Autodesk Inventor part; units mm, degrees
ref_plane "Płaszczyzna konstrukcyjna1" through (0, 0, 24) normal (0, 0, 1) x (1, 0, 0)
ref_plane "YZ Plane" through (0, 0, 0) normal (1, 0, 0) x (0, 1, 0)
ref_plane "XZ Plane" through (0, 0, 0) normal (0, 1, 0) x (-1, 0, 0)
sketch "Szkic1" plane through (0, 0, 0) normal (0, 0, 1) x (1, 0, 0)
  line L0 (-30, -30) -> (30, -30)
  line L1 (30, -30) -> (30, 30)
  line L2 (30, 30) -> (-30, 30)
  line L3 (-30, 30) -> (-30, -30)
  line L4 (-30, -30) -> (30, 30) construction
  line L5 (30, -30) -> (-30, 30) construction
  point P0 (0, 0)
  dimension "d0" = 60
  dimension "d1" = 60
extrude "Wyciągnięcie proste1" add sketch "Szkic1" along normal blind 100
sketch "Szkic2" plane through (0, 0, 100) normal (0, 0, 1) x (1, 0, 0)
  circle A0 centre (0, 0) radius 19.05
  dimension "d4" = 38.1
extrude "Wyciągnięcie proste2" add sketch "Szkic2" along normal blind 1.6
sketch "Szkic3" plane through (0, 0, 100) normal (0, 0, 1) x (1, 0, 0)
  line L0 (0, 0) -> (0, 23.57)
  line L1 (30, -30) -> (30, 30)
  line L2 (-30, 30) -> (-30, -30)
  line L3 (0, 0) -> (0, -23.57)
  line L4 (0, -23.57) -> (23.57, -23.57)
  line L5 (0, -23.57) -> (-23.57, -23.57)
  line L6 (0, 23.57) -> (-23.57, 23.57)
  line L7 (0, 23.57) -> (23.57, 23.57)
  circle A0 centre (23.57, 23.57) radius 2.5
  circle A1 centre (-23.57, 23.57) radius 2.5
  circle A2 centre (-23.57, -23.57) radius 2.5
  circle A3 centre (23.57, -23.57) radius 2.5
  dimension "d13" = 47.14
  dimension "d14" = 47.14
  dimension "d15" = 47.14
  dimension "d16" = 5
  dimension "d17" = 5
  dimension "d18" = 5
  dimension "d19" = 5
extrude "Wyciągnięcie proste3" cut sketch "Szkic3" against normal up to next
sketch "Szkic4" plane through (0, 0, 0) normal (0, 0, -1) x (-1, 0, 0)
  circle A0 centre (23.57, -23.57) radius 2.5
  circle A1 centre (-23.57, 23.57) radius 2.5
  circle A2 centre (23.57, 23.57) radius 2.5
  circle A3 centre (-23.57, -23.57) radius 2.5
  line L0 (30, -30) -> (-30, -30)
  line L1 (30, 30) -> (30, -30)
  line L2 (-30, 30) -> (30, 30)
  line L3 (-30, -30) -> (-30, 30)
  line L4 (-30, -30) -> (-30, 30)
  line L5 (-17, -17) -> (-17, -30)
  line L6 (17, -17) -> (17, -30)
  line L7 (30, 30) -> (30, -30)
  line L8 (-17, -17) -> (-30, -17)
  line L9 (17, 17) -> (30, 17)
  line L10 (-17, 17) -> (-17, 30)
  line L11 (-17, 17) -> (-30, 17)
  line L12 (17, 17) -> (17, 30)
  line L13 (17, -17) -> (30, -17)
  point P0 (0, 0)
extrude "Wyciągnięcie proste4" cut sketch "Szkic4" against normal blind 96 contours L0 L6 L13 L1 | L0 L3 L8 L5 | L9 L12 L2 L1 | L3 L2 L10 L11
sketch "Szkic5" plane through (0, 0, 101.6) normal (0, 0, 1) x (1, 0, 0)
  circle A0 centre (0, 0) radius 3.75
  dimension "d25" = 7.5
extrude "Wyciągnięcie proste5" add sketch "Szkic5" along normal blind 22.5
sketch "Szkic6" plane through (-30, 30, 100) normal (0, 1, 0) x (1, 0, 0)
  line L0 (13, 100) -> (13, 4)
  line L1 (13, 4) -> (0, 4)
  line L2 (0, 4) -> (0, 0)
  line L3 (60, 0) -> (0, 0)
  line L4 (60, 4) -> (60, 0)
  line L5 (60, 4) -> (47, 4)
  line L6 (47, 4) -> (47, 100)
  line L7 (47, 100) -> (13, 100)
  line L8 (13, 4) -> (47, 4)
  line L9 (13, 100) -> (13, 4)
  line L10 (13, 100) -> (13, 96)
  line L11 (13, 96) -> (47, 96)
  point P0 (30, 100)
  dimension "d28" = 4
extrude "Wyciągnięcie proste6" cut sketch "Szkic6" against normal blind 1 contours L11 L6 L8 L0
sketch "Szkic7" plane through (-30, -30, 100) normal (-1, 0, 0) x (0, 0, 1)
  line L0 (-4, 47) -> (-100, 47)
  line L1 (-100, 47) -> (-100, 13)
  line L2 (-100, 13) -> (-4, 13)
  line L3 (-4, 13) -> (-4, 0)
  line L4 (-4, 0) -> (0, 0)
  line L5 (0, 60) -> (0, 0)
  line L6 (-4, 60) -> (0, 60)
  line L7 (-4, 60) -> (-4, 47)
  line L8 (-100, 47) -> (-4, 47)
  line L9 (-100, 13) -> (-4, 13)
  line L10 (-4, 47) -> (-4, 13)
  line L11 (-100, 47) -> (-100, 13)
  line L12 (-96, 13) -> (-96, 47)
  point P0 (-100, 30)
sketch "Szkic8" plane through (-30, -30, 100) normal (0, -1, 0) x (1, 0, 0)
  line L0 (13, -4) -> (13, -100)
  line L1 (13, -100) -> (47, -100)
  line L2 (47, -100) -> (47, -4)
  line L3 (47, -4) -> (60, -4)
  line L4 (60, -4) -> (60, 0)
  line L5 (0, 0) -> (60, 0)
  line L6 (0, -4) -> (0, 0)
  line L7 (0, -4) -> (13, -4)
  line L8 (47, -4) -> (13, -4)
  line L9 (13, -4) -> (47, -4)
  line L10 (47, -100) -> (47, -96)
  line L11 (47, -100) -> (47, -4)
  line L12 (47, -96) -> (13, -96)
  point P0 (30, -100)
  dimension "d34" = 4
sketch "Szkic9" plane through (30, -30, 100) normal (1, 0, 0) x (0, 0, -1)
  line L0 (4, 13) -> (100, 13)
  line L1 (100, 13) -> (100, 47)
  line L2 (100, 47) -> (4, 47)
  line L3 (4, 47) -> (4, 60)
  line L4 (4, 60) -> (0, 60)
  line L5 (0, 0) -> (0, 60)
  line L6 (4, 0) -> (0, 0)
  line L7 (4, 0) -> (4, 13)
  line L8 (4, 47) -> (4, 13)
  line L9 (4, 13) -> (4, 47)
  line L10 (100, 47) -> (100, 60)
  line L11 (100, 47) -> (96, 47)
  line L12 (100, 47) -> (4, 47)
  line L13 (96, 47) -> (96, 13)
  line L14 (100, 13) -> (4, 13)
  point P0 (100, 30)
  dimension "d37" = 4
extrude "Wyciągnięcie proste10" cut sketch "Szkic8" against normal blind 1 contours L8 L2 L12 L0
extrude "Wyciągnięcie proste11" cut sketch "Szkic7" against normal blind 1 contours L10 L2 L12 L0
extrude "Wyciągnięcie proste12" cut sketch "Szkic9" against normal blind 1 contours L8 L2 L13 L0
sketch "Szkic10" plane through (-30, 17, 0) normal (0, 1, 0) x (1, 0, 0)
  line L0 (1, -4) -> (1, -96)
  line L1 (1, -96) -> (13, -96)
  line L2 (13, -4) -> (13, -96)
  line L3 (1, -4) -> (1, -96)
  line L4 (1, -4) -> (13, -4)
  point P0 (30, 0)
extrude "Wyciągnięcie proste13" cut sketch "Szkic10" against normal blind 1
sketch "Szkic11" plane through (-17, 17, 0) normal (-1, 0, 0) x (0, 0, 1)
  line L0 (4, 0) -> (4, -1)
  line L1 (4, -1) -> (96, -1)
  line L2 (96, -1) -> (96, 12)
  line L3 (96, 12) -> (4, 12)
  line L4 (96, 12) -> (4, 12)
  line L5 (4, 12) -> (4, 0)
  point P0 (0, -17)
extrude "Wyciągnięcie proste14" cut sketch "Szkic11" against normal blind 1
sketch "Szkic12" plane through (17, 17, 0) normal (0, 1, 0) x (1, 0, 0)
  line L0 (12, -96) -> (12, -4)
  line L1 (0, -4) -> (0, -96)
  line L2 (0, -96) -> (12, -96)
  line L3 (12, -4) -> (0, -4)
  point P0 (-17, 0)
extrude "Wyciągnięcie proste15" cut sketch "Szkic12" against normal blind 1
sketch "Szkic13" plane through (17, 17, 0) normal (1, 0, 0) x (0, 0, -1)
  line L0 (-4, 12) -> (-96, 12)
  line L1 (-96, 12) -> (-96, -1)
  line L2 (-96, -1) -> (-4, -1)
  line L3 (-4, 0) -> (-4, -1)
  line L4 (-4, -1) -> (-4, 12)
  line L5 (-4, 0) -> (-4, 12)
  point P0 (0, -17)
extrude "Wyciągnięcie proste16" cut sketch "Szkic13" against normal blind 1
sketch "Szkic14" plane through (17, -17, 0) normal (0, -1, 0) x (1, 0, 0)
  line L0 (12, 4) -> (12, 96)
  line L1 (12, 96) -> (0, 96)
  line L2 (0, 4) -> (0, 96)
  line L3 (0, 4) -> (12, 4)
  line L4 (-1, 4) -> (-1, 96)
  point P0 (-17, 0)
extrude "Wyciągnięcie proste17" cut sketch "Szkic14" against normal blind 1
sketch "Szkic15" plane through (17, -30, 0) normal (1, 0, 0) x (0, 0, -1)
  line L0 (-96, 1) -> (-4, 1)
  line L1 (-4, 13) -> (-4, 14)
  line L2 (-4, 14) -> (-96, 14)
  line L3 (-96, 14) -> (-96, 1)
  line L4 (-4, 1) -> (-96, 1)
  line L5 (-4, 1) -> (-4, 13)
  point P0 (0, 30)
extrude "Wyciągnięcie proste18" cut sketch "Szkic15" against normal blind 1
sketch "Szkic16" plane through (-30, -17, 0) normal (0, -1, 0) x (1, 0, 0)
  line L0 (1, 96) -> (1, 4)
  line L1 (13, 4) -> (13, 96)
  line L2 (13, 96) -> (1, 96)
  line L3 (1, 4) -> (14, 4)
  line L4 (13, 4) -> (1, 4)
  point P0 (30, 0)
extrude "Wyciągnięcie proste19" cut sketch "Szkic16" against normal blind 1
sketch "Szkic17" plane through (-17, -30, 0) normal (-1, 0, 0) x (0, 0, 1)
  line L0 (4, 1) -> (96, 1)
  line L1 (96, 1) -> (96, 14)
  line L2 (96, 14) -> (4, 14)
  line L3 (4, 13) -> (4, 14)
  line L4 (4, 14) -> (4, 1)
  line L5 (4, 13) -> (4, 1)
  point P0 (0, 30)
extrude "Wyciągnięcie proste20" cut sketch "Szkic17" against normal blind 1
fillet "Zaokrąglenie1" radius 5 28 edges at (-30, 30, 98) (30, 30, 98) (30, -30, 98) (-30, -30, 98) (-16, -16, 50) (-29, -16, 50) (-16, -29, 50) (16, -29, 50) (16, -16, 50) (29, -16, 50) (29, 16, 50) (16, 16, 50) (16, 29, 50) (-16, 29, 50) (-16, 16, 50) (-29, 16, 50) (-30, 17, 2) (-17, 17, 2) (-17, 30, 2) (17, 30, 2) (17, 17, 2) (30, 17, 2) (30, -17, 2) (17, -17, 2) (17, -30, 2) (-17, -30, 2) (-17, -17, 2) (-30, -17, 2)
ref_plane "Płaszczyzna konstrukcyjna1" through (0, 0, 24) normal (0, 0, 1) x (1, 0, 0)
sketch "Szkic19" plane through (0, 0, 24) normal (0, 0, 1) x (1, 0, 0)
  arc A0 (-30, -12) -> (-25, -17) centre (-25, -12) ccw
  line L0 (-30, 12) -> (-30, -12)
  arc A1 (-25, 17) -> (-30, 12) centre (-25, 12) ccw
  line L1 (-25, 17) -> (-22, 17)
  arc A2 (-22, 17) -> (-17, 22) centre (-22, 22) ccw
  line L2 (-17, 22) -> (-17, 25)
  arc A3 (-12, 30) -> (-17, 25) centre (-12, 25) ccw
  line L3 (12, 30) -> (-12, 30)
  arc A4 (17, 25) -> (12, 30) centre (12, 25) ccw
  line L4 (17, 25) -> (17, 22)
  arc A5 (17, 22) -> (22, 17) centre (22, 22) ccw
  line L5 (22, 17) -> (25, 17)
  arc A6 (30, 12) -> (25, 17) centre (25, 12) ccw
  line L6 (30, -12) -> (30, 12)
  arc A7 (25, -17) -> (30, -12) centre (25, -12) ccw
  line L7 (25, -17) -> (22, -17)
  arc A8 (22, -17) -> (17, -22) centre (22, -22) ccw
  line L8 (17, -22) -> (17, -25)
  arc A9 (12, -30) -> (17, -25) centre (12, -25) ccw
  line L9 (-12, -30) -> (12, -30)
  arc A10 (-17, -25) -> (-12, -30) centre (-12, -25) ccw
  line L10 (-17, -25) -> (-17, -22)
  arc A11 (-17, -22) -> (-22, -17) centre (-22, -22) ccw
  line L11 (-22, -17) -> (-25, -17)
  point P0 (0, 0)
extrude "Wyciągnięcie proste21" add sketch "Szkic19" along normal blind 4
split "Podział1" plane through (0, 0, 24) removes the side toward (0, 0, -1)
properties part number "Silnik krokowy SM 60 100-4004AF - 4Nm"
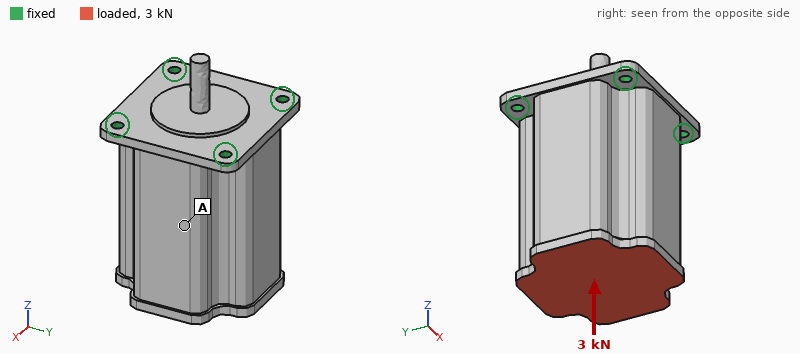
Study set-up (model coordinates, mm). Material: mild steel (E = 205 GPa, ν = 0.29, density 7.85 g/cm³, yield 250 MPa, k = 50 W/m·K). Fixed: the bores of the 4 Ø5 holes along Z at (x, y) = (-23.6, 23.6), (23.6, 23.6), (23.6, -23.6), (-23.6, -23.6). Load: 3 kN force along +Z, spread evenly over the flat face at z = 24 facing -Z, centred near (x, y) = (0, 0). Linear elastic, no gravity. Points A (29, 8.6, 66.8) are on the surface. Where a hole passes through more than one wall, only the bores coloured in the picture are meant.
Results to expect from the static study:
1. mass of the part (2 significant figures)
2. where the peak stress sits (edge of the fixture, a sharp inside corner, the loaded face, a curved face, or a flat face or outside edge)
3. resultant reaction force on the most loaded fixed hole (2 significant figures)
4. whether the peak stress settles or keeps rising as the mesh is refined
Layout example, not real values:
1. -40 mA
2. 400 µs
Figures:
1. 1.6 kg
2. edge of the fixture
3. 810 N
4. keeps rising
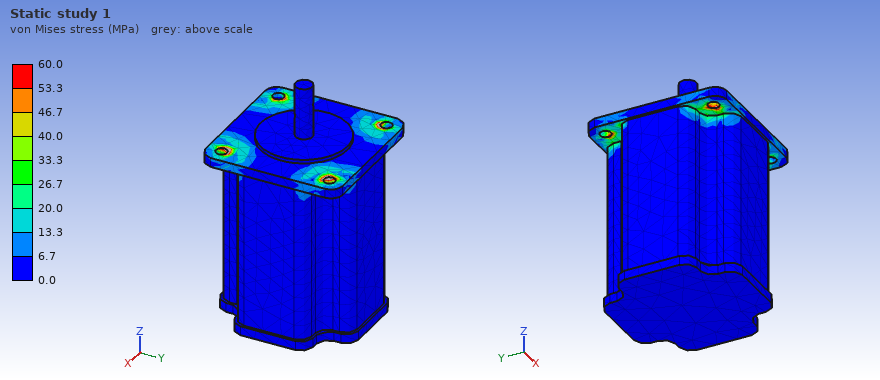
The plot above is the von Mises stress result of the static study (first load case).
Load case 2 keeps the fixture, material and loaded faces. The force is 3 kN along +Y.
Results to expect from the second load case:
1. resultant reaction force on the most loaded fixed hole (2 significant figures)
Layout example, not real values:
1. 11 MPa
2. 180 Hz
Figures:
1. 2.8 kN
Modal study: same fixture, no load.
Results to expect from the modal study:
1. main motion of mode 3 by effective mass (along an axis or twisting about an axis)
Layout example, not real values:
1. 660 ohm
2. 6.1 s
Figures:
1. along Z
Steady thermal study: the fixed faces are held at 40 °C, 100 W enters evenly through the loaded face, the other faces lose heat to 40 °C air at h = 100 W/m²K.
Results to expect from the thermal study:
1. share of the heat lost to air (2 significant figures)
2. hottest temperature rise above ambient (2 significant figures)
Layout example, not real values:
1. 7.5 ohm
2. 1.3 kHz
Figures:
1. 65 %
2. 57 K
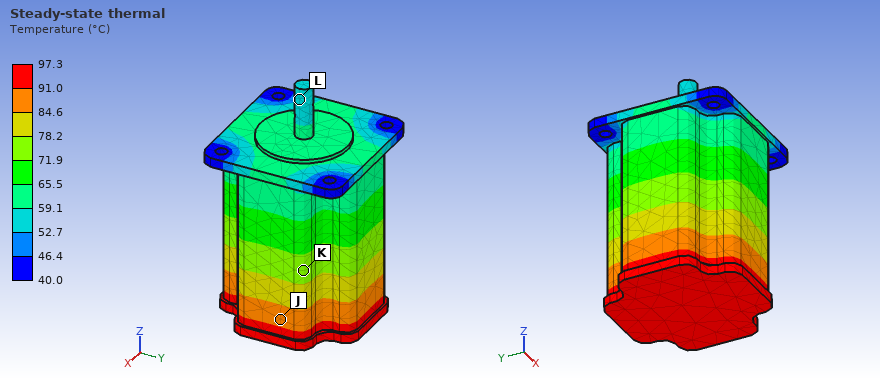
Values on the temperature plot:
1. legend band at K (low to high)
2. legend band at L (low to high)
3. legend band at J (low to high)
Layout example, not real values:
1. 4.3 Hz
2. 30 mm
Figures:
1. 71.9 to 78.2 °C
2. 52.7 to 59.1 °C
3. 84.6 to 91.0 °C
